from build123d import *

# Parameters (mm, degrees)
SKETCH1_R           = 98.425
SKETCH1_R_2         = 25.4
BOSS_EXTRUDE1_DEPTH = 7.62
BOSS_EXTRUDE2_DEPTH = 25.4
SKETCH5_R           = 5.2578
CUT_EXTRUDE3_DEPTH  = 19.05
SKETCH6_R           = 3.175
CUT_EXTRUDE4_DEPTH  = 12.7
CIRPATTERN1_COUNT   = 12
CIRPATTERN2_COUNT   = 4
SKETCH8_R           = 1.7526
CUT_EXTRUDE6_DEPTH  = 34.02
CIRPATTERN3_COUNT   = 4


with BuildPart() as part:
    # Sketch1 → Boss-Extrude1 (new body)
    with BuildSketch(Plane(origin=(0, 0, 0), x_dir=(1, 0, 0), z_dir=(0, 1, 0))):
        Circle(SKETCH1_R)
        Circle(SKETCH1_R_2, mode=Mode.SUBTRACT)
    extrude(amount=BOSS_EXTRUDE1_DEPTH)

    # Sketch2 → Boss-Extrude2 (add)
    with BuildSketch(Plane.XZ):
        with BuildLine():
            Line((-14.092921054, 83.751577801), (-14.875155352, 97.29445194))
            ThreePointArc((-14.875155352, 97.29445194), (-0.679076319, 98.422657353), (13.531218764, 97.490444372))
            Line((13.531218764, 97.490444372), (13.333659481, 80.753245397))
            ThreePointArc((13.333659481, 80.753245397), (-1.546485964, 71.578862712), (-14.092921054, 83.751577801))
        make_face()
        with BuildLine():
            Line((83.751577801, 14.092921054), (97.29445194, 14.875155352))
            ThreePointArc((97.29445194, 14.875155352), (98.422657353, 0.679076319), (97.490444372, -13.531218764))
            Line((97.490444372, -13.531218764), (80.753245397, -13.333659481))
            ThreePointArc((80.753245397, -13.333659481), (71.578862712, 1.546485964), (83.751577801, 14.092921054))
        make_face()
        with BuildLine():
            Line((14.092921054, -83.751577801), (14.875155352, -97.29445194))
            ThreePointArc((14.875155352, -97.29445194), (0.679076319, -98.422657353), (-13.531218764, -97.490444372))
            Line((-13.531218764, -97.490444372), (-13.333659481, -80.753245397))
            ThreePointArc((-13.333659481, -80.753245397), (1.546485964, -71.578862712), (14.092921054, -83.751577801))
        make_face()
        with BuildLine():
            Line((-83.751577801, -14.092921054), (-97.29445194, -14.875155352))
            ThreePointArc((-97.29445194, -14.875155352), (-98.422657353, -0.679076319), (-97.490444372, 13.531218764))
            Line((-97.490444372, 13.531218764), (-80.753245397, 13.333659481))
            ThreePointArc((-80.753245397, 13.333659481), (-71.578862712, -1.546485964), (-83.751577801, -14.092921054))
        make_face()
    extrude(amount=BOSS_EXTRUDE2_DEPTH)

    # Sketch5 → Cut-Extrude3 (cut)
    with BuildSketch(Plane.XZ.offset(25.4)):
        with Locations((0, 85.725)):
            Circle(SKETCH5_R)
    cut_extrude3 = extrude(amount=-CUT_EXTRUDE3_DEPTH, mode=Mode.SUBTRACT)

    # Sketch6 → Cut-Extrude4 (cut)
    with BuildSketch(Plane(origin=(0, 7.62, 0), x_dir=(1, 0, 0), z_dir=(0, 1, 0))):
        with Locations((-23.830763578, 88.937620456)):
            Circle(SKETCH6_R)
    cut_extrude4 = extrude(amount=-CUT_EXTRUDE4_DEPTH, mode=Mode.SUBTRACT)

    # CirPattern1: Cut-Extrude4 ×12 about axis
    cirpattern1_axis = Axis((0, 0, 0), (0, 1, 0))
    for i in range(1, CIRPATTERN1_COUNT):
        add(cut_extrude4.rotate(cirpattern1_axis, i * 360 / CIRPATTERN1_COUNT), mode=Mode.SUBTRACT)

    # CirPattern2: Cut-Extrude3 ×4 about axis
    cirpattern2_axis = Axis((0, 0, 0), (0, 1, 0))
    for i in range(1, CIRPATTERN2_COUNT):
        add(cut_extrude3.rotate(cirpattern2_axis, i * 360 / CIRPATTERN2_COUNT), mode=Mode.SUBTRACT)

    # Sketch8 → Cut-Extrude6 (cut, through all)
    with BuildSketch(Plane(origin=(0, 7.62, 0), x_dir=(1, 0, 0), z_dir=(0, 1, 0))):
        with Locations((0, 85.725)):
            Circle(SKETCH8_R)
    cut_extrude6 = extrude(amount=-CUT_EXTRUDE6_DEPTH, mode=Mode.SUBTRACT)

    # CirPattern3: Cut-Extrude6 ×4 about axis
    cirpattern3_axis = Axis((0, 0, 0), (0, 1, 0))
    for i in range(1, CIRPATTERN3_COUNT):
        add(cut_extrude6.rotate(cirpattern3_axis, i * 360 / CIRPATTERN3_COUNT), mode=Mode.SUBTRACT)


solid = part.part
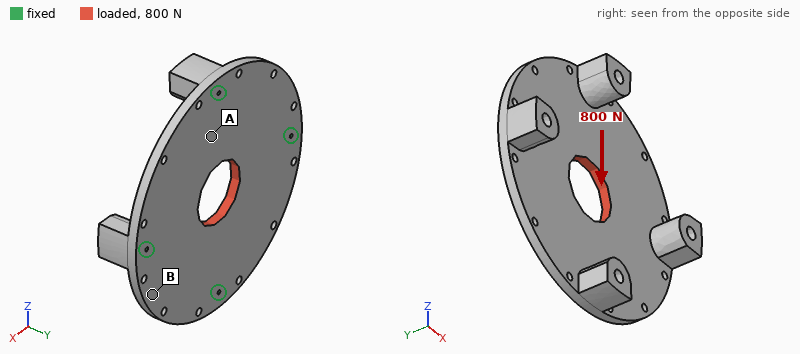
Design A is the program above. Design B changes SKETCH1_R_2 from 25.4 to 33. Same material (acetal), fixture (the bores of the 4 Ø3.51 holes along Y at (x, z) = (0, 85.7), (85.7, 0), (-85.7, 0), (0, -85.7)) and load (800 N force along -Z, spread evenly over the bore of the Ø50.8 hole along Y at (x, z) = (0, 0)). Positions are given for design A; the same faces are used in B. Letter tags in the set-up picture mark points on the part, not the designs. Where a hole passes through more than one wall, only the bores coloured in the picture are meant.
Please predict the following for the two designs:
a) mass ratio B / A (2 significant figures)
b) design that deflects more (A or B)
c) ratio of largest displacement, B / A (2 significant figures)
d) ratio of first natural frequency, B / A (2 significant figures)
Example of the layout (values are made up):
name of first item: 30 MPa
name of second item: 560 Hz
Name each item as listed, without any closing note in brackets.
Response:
mass ratio B / A: 0.96
design that deflects more: A
ratio of largest displacement, B / A: 0.92
ratio of first natural frequency, B / A: 1.0
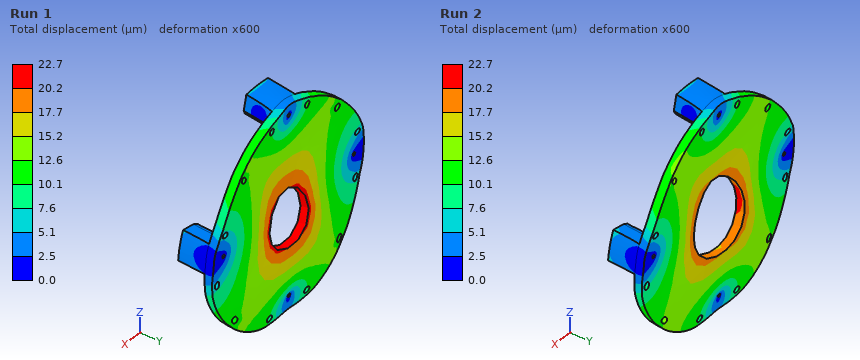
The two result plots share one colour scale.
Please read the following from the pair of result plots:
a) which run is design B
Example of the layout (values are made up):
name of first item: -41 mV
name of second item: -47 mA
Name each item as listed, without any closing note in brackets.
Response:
which run is design B: Run 2
